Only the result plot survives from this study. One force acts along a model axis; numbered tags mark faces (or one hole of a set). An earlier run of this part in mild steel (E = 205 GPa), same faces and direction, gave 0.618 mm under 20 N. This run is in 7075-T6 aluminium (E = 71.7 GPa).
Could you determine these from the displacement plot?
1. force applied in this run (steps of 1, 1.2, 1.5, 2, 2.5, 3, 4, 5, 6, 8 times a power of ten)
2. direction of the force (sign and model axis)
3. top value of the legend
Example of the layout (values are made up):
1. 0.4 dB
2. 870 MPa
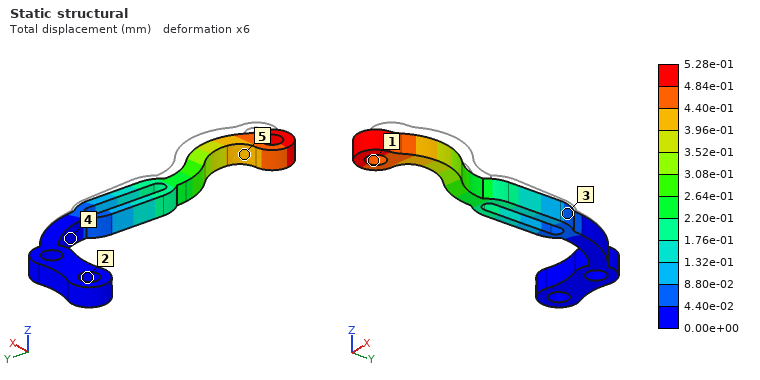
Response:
1. 6 N
2. -X
3. 5.28e-01 mm
